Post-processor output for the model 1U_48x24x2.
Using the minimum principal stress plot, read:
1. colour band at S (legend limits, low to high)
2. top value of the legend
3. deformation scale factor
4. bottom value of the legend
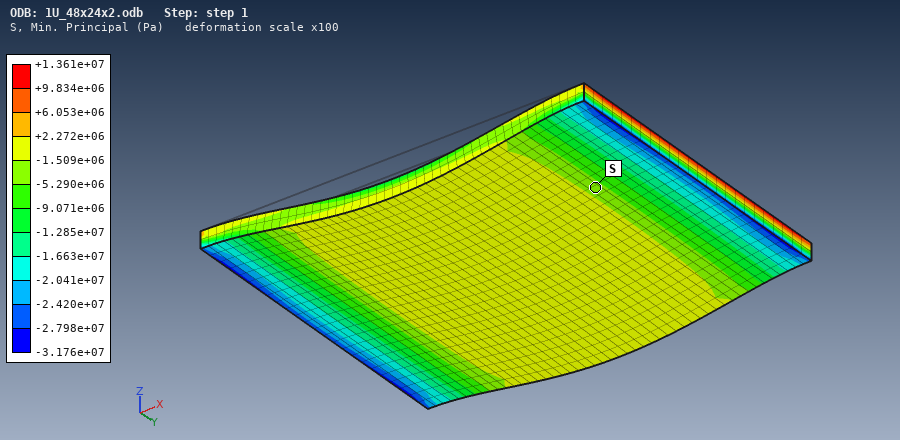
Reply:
-5.290e+06 to -1.509e+06 Pa
+1.361e+07 Pa
100
-3.176e+07 Pa
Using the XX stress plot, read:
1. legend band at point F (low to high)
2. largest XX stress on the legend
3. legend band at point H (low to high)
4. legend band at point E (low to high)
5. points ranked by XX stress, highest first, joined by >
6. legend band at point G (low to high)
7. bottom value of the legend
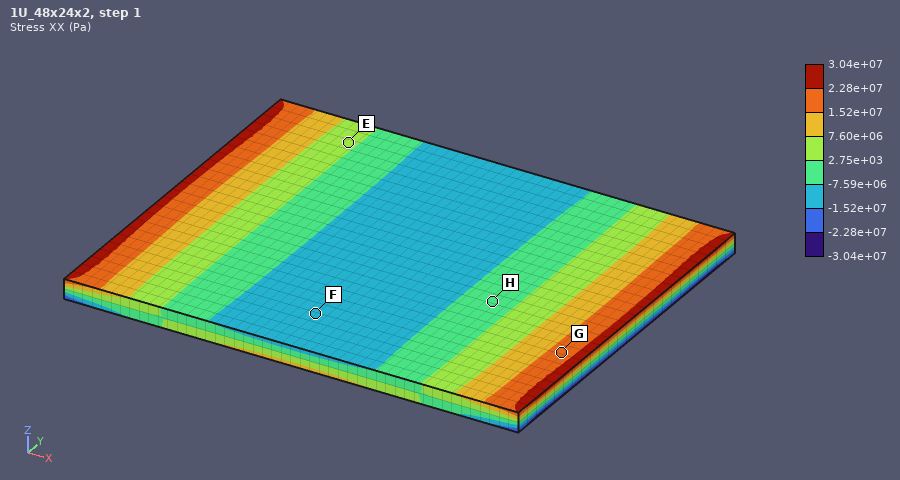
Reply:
-1.52e+07 to -7.59e+06 Pa
3.04e+07 Pa
-7.59e+06 to 2.75e+03 Pa
2.75e+03 to 7.60e+06 Pa
G > E > H > F
1.52e+07 to 2.28e+07 Pa
-3.04e+07 Pa
